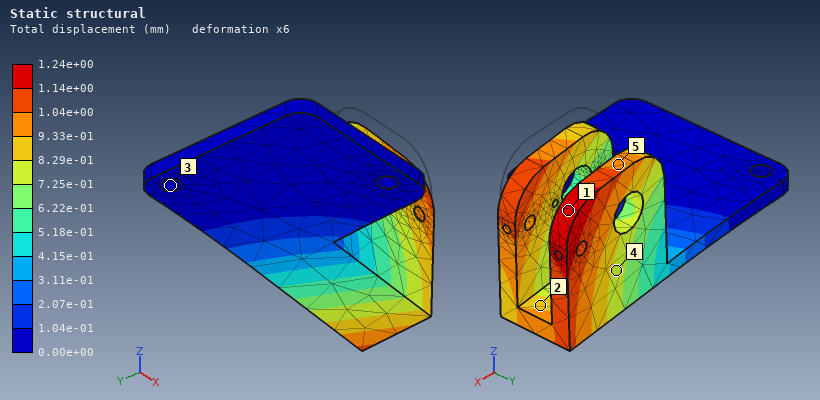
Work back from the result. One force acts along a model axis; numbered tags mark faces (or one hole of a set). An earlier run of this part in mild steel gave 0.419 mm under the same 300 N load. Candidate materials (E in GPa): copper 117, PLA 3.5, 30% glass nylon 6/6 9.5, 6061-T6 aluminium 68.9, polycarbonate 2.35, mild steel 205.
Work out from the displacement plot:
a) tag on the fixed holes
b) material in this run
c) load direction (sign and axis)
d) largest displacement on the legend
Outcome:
3
6061-T6 aluminium
-Z
1.24e+00 mm
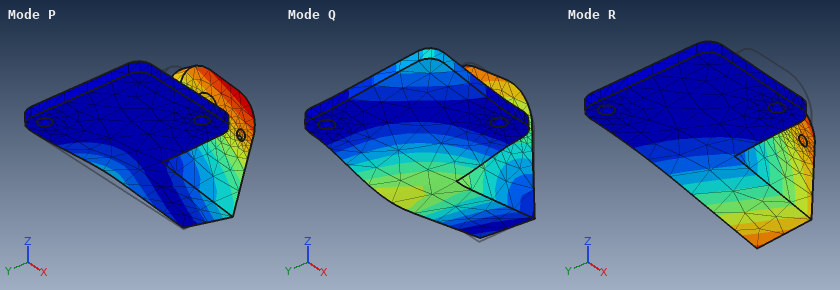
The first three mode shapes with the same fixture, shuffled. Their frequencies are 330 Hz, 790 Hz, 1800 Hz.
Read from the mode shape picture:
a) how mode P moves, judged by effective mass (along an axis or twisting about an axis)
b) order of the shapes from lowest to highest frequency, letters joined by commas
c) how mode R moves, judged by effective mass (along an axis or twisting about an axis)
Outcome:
along Y
R, P, Q
along Z
